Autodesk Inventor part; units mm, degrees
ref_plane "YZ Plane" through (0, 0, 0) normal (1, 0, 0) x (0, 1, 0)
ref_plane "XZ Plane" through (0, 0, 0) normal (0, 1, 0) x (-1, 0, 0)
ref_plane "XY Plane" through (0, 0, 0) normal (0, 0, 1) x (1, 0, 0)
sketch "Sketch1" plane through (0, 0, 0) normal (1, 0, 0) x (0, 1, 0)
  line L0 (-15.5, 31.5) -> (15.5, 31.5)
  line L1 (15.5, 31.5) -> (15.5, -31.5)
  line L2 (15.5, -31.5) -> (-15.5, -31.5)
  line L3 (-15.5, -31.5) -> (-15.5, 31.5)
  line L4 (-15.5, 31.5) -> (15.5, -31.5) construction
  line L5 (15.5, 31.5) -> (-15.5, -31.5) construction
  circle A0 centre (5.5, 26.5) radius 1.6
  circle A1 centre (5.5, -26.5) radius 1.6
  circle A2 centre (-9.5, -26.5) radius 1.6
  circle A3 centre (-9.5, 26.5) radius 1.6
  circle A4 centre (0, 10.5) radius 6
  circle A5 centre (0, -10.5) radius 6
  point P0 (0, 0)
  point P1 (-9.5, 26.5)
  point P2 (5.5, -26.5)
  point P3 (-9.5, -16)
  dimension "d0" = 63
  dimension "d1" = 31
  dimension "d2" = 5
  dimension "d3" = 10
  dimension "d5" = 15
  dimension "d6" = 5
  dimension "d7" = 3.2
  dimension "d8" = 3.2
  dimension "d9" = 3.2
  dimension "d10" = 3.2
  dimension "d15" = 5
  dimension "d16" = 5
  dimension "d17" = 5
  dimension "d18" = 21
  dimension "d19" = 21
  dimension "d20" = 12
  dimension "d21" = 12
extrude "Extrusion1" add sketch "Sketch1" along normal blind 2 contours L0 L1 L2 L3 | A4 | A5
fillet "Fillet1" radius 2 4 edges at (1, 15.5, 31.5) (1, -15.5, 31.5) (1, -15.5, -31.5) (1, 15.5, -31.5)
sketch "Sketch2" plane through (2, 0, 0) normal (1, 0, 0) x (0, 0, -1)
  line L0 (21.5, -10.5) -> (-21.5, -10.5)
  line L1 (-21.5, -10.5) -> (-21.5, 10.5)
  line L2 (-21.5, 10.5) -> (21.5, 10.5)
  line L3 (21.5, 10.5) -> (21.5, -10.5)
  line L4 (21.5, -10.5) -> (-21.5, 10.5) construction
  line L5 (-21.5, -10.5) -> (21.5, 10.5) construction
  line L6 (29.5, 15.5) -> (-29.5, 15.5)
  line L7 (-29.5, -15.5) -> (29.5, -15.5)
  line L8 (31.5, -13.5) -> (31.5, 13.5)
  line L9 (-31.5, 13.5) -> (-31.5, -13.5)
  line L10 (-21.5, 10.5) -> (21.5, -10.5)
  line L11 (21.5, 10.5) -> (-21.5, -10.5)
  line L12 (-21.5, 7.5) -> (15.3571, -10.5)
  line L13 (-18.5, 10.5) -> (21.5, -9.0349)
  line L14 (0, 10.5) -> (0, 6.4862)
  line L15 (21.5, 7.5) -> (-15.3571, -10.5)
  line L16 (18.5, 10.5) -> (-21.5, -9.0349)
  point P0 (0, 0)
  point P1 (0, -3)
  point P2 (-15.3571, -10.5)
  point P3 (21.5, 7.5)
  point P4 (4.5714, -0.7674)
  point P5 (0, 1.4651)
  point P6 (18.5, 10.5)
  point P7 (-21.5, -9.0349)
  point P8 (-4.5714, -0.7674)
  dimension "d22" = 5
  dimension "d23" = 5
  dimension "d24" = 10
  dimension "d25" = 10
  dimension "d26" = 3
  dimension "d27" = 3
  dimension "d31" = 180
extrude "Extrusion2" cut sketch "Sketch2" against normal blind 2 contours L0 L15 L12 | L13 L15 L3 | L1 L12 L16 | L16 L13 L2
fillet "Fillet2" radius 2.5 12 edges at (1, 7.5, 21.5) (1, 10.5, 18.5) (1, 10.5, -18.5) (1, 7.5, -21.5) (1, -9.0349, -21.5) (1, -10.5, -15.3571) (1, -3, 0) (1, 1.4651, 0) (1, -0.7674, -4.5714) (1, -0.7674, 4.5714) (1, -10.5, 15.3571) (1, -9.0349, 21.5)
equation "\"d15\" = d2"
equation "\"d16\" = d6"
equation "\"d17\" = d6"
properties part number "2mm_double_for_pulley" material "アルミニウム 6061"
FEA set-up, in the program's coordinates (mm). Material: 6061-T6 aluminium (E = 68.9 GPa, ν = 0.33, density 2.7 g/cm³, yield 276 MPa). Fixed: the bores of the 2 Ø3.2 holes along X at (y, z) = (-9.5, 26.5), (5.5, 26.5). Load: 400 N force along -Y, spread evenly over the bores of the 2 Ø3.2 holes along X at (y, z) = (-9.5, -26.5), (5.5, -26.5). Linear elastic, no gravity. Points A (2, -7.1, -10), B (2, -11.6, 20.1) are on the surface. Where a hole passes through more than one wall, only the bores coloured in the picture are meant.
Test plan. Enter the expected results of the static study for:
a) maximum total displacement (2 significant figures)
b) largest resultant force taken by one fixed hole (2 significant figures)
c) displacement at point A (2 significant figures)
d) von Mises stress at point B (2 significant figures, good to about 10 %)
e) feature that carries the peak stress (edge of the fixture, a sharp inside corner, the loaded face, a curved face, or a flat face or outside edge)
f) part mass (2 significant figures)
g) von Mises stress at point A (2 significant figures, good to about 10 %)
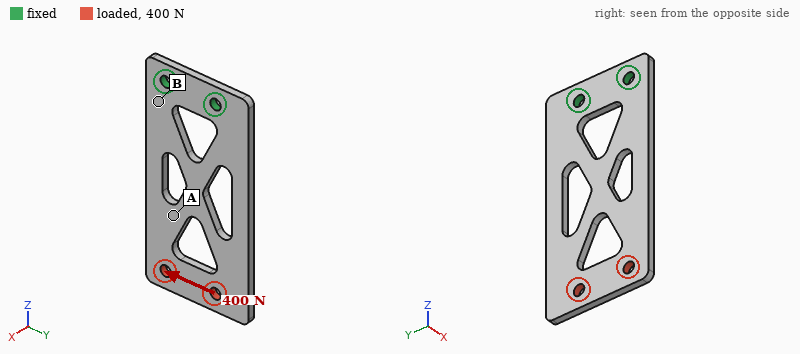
0.19 mm
1.1 kN
0.11 mm
69 MPa
edge of the fixture
7.9 g
28 MPa
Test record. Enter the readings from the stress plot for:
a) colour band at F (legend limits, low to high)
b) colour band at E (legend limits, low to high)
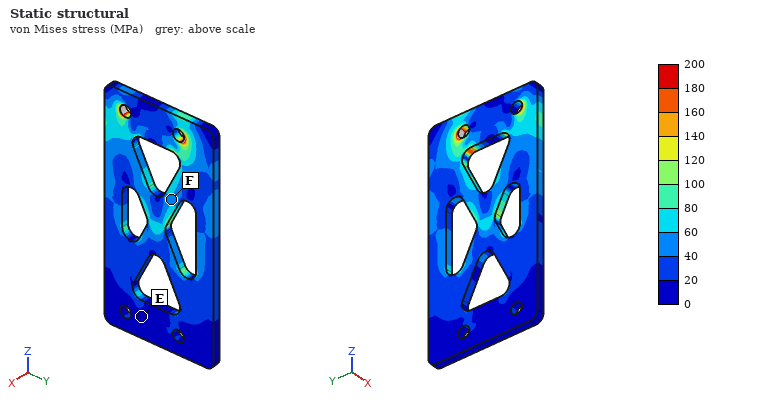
40 to 60 MPa
0 to 20 MPa
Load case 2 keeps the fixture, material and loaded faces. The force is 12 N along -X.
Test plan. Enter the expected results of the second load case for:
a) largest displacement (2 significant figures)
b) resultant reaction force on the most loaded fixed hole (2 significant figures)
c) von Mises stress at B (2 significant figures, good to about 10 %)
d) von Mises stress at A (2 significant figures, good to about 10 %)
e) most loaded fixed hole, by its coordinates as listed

0.76 mm
7.1 N
47 MPa
12 MPa
(-9.5, 26.5)
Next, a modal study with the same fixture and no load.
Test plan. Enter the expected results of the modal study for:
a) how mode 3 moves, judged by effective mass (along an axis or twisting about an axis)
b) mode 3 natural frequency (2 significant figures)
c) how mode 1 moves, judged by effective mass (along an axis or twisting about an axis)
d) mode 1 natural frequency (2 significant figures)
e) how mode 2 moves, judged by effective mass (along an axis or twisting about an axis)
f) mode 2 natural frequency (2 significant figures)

along X
2800 Hz
along X
430 Hz
twisting about Z
1600 Hz
